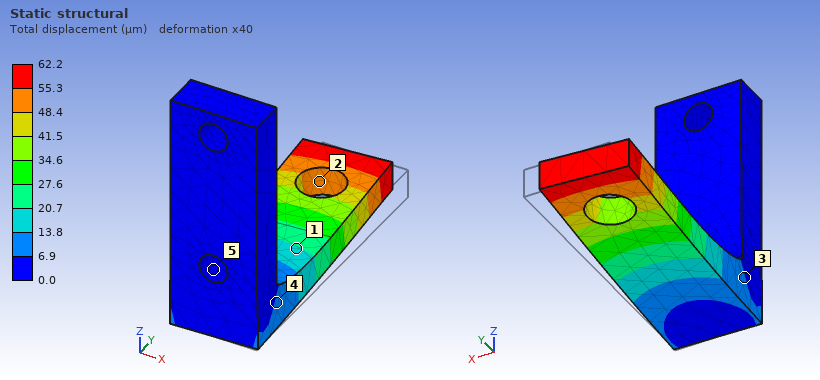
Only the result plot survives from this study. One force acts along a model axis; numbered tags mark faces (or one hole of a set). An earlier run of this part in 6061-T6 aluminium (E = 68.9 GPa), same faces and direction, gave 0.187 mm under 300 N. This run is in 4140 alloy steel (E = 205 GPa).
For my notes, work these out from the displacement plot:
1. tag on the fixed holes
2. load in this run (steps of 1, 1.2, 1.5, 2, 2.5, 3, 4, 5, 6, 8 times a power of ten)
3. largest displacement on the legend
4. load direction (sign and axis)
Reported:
5
300 N
62.2 µm
-X
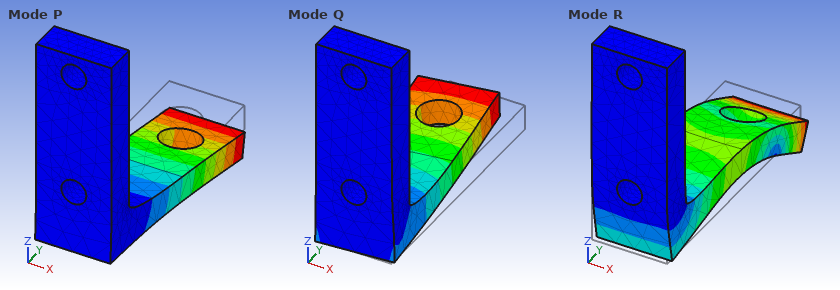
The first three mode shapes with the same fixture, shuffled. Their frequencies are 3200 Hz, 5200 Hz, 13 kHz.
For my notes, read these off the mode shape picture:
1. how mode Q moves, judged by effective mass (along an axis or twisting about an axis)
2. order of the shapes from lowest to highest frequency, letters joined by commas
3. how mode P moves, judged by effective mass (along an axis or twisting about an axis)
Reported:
along X
P, Q, R
along Z
